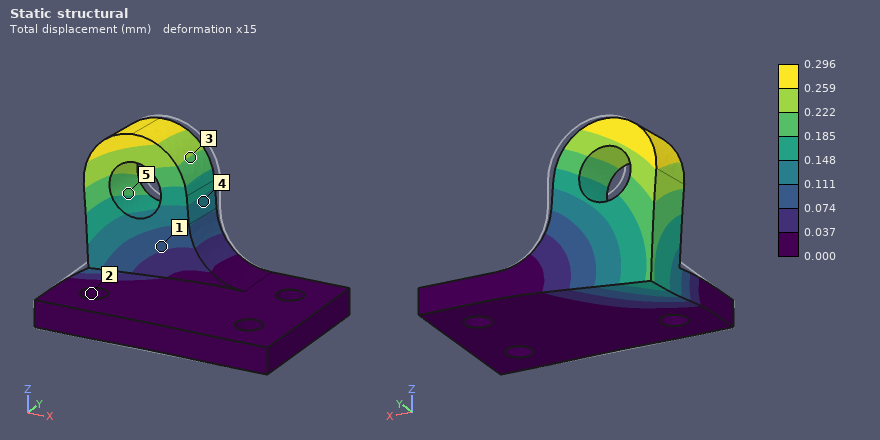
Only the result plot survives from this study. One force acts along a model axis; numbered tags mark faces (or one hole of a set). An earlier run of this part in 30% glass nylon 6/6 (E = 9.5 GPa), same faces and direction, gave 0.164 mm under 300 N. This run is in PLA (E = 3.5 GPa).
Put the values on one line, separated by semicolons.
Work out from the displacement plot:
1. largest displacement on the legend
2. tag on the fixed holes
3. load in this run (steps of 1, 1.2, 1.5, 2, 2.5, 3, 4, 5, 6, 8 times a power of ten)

0.296 mm; 2; 200 N
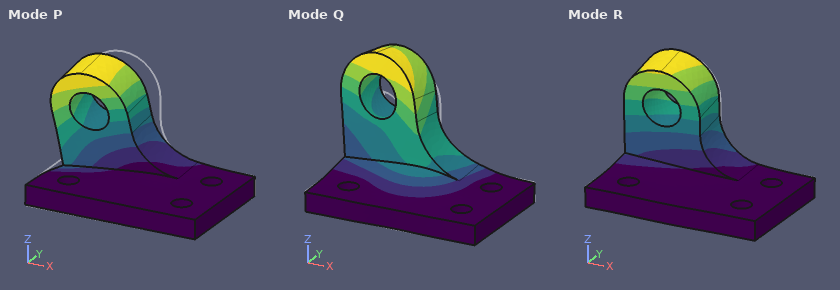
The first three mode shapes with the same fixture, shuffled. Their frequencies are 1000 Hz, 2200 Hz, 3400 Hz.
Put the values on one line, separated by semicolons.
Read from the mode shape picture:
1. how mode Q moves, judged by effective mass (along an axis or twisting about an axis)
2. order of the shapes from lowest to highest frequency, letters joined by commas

along Z; R, P, Q
